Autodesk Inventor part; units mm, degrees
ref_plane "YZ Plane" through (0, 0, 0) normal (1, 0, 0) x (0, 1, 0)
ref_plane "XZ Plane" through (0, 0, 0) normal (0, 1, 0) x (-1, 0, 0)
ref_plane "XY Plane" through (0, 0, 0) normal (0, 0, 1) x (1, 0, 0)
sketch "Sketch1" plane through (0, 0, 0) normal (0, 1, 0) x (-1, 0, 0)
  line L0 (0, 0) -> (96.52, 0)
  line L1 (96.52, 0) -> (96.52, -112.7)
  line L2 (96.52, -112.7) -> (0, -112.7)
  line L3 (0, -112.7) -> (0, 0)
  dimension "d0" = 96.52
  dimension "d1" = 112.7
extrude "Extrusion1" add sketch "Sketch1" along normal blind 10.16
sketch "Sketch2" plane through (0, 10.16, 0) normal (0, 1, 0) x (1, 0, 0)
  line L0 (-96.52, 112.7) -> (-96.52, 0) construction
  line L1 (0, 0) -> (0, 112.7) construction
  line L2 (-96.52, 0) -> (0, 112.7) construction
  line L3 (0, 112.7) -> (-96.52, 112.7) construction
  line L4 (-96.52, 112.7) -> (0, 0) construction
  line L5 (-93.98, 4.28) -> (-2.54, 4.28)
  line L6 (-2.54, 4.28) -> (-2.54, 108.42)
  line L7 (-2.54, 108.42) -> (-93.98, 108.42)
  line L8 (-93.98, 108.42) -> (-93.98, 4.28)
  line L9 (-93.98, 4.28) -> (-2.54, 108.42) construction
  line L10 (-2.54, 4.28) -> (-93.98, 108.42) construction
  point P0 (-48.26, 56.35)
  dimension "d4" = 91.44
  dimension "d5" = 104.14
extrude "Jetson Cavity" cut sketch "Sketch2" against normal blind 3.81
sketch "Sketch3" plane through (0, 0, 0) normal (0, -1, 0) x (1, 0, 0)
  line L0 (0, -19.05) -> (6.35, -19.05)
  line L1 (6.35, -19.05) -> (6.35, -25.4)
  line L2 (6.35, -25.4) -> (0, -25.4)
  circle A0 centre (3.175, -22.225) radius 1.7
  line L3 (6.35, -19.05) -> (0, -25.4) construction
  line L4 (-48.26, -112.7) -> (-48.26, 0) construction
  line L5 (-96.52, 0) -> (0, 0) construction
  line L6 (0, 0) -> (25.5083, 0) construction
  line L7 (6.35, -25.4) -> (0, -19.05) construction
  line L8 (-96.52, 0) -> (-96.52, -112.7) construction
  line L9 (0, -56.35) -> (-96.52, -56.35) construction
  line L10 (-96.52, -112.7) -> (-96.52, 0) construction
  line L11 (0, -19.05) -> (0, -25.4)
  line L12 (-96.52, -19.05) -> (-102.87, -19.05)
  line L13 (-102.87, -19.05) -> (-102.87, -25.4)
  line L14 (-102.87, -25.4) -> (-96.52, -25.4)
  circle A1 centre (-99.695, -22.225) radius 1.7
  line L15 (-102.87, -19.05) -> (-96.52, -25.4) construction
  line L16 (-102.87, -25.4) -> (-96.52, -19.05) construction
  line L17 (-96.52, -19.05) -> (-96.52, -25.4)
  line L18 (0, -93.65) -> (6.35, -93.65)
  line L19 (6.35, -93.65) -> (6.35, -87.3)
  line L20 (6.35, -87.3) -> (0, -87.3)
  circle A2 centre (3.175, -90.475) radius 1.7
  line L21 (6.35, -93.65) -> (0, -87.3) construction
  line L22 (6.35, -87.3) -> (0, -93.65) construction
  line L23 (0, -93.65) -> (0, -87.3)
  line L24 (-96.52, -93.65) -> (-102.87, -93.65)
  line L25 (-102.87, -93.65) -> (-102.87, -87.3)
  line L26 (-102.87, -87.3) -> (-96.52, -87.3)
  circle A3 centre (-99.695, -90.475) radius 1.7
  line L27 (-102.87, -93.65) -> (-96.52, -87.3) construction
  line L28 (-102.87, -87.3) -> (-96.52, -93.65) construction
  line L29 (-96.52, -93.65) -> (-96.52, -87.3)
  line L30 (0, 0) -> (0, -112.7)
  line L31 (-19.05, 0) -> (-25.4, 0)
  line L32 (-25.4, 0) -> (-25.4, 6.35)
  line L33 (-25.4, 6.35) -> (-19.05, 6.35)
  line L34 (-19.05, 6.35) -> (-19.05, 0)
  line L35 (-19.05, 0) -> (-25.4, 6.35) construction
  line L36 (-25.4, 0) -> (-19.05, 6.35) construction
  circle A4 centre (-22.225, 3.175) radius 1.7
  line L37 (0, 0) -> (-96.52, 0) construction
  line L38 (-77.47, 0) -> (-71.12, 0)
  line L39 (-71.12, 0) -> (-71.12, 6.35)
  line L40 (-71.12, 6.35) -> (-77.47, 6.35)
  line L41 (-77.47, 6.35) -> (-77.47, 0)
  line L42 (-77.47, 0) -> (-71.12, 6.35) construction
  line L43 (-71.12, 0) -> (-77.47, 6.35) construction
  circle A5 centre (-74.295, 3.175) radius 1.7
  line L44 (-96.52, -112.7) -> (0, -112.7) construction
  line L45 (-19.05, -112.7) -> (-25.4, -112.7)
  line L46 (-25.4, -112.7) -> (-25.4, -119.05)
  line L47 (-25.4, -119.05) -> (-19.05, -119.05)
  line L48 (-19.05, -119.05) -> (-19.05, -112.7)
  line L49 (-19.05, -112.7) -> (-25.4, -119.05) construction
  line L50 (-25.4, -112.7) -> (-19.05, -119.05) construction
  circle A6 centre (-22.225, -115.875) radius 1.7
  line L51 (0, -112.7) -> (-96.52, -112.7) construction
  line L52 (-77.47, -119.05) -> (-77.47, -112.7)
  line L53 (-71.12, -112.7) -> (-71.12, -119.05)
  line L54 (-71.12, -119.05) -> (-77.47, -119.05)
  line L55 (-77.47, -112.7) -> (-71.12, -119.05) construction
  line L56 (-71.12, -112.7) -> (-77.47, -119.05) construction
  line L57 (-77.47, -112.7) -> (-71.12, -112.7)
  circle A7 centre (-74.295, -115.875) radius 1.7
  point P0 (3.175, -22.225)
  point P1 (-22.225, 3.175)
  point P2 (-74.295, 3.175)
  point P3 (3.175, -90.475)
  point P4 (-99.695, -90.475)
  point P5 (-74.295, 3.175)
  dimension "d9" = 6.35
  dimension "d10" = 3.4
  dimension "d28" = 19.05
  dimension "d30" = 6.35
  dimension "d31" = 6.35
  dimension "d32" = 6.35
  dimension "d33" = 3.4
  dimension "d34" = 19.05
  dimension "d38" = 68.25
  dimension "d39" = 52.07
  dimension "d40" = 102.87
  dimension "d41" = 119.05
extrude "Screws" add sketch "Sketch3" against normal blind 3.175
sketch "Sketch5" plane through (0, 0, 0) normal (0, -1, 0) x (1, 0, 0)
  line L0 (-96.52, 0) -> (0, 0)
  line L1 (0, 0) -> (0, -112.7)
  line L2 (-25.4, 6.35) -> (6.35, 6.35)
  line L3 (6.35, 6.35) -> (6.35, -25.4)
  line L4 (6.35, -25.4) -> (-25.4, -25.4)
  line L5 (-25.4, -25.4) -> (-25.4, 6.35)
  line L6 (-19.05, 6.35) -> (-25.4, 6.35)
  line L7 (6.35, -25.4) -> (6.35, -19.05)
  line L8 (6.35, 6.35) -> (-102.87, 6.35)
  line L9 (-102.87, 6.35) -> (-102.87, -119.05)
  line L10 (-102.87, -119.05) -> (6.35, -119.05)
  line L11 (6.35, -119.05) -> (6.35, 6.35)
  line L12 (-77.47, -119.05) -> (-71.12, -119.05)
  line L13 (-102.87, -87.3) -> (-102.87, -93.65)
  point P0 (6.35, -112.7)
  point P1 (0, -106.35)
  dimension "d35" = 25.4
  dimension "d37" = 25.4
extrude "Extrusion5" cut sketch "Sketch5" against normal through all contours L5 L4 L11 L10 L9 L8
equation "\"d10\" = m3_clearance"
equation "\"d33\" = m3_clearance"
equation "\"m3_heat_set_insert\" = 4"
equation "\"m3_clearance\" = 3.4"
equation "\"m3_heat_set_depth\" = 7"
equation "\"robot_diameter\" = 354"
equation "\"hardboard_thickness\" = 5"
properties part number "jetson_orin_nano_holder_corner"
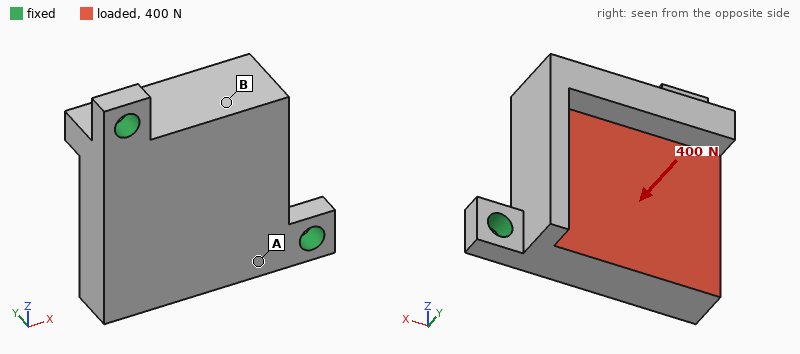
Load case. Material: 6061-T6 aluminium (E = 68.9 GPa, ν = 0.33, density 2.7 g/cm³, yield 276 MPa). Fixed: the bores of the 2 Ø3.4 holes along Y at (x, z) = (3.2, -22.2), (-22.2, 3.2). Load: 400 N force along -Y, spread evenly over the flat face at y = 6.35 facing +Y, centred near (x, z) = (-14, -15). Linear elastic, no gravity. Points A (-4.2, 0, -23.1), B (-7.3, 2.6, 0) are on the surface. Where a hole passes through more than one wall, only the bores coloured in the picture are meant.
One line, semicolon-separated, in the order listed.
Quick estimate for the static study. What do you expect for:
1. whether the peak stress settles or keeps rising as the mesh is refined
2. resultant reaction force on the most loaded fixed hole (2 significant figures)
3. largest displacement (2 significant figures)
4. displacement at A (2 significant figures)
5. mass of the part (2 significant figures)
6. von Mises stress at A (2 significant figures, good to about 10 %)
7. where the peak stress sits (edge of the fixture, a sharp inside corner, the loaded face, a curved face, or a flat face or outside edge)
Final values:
keeps rising; 240 N; 71 µm; 15 µm; 13 g; 17 MPa; edge of the fixture
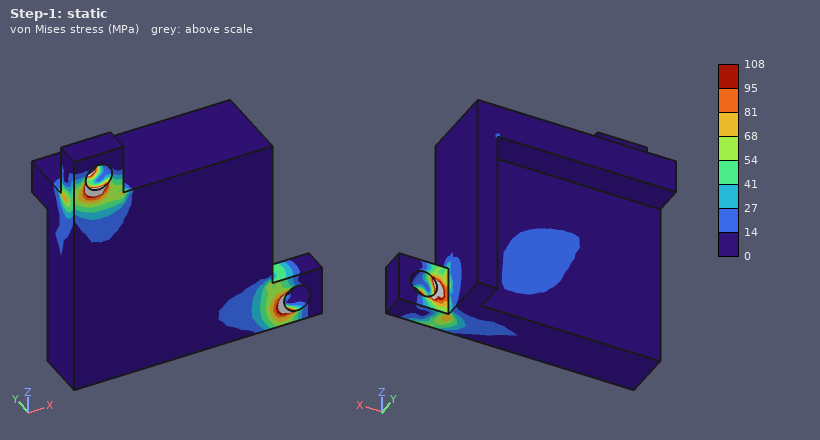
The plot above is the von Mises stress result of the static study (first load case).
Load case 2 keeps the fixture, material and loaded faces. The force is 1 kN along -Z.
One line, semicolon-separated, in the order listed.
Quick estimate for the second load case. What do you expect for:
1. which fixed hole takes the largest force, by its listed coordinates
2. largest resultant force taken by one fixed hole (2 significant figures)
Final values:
(-22.2, 3.2); 690 N
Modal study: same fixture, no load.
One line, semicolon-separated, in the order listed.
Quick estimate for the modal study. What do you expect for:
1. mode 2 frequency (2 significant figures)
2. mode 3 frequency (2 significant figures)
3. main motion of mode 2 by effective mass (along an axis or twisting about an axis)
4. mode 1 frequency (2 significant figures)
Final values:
10 kHz; 20 kHz; along Y; 4600 Hz
